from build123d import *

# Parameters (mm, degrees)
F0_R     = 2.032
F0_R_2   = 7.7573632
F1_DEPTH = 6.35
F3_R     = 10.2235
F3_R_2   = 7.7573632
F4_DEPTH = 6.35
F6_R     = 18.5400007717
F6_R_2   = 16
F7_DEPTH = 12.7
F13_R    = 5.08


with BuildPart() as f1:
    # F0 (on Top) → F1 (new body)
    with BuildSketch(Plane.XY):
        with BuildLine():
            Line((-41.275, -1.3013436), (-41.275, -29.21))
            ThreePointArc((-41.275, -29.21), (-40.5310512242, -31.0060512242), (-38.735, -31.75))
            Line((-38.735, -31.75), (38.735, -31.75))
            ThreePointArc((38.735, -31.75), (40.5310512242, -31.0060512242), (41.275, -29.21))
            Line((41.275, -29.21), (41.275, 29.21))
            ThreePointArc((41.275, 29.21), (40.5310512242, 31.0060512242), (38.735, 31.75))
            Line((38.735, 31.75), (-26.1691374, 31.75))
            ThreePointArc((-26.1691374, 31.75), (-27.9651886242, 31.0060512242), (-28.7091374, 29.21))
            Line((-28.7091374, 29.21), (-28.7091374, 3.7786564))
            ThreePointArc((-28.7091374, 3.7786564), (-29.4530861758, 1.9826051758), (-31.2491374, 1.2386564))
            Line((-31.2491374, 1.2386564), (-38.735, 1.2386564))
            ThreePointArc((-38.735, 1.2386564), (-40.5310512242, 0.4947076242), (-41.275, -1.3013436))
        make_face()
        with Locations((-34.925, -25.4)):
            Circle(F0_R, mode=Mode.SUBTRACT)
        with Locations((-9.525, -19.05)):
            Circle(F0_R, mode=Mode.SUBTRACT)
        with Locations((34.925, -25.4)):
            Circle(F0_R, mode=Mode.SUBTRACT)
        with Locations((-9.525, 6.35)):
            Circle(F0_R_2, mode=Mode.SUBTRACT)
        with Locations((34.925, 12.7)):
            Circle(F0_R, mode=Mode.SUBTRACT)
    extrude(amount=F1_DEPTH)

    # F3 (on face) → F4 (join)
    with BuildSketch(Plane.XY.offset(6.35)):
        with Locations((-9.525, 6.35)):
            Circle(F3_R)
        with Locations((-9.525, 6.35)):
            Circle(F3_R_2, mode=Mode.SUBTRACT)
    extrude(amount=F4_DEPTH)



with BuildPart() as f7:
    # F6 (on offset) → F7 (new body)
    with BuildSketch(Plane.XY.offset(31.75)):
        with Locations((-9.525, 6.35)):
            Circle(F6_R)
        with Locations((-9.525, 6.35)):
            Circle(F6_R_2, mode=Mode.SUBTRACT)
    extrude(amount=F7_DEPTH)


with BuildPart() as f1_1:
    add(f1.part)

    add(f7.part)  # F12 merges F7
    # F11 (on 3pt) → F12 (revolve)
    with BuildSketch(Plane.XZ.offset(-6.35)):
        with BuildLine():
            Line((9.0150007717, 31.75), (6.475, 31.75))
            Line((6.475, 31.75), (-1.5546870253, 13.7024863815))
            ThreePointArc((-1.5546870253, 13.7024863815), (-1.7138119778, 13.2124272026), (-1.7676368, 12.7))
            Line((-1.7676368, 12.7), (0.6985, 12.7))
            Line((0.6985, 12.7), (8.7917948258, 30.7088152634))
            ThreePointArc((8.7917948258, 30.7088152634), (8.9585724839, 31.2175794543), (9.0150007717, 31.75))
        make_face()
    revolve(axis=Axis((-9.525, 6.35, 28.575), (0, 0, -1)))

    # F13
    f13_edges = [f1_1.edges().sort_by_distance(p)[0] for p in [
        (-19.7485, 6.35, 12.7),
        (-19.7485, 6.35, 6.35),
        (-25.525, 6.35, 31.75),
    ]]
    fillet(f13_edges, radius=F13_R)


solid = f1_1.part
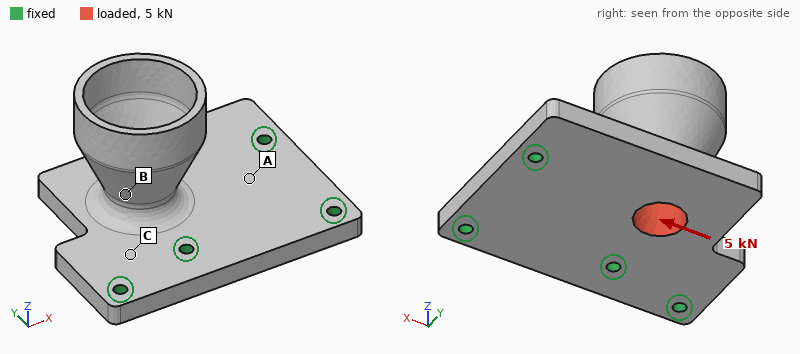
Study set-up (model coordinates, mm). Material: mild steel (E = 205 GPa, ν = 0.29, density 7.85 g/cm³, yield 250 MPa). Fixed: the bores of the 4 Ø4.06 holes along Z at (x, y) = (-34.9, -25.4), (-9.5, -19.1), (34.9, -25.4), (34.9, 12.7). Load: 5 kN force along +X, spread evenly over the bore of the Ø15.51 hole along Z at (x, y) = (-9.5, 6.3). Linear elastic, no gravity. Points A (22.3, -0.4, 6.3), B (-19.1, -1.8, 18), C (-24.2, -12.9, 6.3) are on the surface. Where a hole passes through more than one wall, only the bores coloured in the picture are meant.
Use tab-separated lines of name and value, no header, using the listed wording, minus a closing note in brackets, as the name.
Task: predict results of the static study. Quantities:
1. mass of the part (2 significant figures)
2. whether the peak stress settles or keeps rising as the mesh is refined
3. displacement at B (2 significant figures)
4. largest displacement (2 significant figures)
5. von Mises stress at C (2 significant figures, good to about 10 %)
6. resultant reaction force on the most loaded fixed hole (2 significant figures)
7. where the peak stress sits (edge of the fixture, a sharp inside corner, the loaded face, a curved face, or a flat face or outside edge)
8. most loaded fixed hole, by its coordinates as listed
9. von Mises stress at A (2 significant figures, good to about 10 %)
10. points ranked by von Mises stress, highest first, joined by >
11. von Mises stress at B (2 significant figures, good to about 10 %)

mass of the part	300 g
whether the peak stress settles or keeps rising as the mesh is refined	keeps rising
displacement at B	11 µm
largest displacement	25 µm
von Mises stress at C	21 MPa
resultant reaction force on the most loaded fixed hole	2.1 kN
where the peak stress sits	edge of the fixture
most loaded fixed hole, by its coordinates as listed	(34.9, 12.7)
von Mises stress at A	9.4 MPa
points ranked by von Mises stress, highest first, joined by >	C > A > B
von Mises stress at B	4.9 MPa
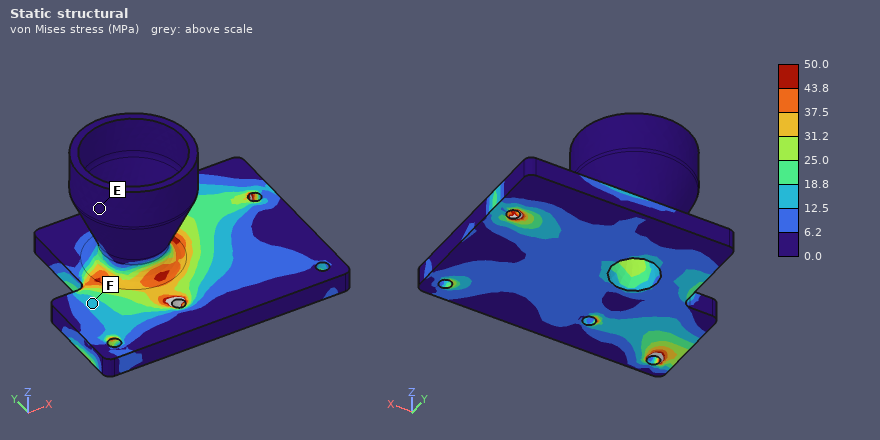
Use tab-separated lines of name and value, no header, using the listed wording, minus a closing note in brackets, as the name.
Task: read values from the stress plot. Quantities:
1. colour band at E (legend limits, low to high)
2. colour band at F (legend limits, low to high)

colour band at E	0.0 to 6.2 MPa
colour band at F	12.5 to 18.8 MPa
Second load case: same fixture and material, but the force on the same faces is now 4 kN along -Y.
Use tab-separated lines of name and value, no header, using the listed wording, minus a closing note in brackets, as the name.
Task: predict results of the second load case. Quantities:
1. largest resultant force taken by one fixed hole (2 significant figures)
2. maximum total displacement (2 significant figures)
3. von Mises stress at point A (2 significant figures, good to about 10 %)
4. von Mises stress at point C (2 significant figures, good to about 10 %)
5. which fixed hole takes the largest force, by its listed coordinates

largest resultant force taken by one fixed hole	2.3 kN
maximum total displacement	34 µm
von Mises stress at point A	15 MPa
von Mises stress at point C	23 MPa
which fixed hole takes the largest force, by its listed coordinates	(-9.5, -19.1)
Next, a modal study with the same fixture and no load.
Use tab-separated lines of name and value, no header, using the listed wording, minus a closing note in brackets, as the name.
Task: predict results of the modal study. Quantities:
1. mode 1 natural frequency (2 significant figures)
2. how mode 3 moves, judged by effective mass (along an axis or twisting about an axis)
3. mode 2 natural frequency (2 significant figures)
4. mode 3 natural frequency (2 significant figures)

mode 1 natural frequency	1900 Hz
how mode 3 moves, judged by effective mass	along Z
mode 2 natural frequency	3400 Hz
mode 3 natural frequency	5800 Hz
